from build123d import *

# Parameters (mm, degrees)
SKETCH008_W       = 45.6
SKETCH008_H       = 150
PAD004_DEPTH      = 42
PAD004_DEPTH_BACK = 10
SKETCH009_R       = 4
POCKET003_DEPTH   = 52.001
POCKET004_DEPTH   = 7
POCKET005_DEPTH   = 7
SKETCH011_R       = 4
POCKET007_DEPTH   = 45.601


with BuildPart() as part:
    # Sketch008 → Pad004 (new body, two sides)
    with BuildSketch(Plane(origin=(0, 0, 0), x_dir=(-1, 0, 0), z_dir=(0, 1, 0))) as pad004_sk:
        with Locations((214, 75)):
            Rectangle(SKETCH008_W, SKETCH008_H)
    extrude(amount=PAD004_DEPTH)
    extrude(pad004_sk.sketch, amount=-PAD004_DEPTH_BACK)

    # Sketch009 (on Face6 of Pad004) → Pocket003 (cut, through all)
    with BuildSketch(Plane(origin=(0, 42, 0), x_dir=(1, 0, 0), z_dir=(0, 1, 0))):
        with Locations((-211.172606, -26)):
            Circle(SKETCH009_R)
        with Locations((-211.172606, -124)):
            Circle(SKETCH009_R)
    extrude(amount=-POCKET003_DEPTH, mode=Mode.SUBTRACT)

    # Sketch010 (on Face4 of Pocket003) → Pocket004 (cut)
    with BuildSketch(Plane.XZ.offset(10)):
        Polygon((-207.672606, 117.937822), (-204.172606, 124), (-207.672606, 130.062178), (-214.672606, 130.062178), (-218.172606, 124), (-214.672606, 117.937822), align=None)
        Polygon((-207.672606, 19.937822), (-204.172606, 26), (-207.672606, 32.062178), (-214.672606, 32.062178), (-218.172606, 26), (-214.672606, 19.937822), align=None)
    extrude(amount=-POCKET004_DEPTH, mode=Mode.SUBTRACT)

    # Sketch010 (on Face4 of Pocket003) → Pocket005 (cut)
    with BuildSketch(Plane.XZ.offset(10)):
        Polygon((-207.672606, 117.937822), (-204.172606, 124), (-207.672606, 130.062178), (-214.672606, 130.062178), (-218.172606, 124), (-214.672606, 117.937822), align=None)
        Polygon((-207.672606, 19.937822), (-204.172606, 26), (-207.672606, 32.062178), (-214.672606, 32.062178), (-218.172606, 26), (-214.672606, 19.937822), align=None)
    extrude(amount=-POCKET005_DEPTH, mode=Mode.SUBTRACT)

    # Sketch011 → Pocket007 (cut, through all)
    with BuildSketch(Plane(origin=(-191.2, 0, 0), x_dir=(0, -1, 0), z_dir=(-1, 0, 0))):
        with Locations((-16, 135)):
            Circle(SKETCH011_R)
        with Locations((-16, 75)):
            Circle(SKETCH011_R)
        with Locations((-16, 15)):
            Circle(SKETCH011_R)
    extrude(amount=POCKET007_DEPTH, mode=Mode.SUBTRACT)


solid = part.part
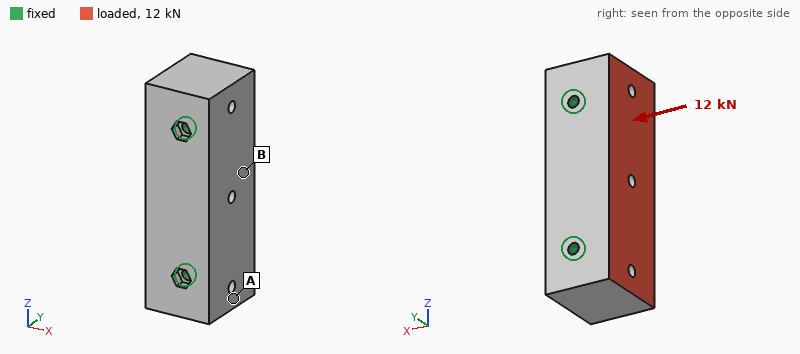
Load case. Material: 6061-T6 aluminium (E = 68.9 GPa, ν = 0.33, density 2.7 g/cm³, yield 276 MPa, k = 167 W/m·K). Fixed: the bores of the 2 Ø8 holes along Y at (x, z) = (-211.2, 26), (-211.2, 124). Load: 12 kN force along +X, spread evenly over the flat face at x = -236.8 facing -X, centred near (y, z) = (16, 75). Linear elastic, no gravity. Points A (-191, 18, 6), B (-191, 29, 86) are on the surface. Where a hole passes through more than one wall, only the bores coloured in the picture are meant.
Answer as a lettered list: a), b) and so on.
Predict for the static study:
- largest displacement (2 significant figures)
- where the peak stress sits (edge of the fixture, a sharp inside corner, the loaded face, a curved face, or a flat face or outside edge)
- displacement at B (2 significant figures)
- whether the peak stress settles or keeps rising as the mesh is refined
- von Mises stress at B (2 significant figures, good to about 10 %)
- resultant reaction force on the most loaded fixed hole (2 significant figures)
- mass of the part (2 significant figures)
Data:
a) 4.5 µm
b) edge of the fixture
c) 3.0 µm
d) keeps rising
e) 3.1 MPa
f) 6.0 kN
g) 920 g
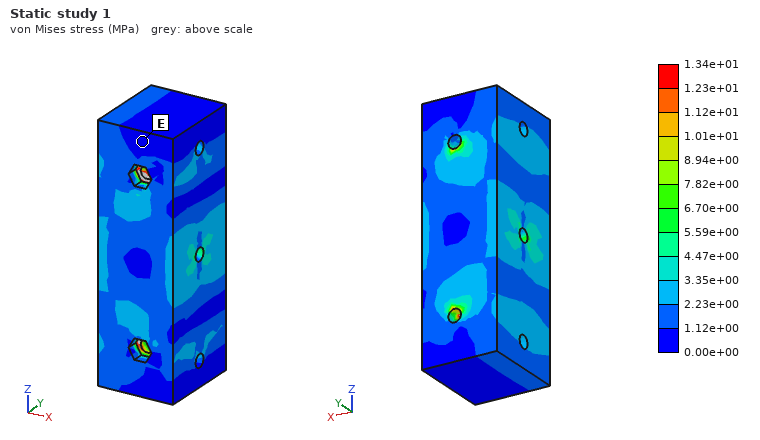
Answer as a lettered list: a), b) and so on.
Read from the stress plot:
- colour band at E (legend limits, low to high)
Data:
a) 0.00e+00 to 1.12e+00 MPa
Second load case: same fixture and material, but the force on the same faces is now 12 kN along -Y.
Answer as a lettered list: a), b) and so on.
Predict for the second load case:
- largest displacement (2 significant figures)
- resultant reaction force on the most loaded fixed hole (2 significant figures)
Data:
a) 11 µm
b) 6.0 kN
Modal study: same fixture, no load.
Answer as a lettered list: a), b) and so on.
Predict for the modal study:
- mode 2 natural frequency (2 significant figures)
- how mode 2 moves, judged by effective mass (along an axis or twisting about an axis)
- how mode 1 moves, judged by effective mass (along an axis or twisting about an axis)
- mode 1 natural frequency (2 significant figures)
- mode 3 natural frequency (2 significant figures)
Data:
a) 11 kHz
b) along Y
c) along X
d) 8800 Hz
e) 12 kHz
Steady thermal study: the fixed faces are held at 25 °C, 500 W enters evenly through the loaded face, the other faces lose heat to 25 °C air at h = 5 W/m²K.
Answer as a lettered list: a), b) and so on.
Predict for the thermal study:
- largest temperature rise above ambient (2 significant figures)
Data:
a) 21 K
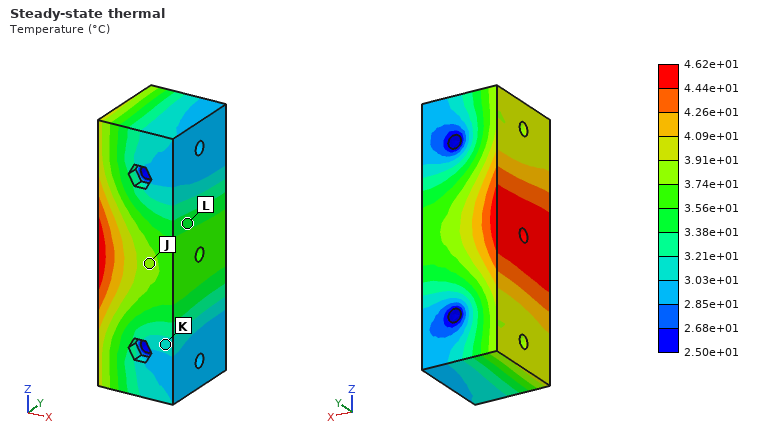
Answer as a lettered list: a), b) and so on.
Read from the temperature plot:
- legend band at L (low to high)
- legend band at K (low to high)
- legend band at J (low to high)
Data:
a) 3.38e+01 to 3.56e+01 °C
b) 3.03e+01 to 3.21e+01 °C
c) 3.74e+01 to 3.91e+01 °C
